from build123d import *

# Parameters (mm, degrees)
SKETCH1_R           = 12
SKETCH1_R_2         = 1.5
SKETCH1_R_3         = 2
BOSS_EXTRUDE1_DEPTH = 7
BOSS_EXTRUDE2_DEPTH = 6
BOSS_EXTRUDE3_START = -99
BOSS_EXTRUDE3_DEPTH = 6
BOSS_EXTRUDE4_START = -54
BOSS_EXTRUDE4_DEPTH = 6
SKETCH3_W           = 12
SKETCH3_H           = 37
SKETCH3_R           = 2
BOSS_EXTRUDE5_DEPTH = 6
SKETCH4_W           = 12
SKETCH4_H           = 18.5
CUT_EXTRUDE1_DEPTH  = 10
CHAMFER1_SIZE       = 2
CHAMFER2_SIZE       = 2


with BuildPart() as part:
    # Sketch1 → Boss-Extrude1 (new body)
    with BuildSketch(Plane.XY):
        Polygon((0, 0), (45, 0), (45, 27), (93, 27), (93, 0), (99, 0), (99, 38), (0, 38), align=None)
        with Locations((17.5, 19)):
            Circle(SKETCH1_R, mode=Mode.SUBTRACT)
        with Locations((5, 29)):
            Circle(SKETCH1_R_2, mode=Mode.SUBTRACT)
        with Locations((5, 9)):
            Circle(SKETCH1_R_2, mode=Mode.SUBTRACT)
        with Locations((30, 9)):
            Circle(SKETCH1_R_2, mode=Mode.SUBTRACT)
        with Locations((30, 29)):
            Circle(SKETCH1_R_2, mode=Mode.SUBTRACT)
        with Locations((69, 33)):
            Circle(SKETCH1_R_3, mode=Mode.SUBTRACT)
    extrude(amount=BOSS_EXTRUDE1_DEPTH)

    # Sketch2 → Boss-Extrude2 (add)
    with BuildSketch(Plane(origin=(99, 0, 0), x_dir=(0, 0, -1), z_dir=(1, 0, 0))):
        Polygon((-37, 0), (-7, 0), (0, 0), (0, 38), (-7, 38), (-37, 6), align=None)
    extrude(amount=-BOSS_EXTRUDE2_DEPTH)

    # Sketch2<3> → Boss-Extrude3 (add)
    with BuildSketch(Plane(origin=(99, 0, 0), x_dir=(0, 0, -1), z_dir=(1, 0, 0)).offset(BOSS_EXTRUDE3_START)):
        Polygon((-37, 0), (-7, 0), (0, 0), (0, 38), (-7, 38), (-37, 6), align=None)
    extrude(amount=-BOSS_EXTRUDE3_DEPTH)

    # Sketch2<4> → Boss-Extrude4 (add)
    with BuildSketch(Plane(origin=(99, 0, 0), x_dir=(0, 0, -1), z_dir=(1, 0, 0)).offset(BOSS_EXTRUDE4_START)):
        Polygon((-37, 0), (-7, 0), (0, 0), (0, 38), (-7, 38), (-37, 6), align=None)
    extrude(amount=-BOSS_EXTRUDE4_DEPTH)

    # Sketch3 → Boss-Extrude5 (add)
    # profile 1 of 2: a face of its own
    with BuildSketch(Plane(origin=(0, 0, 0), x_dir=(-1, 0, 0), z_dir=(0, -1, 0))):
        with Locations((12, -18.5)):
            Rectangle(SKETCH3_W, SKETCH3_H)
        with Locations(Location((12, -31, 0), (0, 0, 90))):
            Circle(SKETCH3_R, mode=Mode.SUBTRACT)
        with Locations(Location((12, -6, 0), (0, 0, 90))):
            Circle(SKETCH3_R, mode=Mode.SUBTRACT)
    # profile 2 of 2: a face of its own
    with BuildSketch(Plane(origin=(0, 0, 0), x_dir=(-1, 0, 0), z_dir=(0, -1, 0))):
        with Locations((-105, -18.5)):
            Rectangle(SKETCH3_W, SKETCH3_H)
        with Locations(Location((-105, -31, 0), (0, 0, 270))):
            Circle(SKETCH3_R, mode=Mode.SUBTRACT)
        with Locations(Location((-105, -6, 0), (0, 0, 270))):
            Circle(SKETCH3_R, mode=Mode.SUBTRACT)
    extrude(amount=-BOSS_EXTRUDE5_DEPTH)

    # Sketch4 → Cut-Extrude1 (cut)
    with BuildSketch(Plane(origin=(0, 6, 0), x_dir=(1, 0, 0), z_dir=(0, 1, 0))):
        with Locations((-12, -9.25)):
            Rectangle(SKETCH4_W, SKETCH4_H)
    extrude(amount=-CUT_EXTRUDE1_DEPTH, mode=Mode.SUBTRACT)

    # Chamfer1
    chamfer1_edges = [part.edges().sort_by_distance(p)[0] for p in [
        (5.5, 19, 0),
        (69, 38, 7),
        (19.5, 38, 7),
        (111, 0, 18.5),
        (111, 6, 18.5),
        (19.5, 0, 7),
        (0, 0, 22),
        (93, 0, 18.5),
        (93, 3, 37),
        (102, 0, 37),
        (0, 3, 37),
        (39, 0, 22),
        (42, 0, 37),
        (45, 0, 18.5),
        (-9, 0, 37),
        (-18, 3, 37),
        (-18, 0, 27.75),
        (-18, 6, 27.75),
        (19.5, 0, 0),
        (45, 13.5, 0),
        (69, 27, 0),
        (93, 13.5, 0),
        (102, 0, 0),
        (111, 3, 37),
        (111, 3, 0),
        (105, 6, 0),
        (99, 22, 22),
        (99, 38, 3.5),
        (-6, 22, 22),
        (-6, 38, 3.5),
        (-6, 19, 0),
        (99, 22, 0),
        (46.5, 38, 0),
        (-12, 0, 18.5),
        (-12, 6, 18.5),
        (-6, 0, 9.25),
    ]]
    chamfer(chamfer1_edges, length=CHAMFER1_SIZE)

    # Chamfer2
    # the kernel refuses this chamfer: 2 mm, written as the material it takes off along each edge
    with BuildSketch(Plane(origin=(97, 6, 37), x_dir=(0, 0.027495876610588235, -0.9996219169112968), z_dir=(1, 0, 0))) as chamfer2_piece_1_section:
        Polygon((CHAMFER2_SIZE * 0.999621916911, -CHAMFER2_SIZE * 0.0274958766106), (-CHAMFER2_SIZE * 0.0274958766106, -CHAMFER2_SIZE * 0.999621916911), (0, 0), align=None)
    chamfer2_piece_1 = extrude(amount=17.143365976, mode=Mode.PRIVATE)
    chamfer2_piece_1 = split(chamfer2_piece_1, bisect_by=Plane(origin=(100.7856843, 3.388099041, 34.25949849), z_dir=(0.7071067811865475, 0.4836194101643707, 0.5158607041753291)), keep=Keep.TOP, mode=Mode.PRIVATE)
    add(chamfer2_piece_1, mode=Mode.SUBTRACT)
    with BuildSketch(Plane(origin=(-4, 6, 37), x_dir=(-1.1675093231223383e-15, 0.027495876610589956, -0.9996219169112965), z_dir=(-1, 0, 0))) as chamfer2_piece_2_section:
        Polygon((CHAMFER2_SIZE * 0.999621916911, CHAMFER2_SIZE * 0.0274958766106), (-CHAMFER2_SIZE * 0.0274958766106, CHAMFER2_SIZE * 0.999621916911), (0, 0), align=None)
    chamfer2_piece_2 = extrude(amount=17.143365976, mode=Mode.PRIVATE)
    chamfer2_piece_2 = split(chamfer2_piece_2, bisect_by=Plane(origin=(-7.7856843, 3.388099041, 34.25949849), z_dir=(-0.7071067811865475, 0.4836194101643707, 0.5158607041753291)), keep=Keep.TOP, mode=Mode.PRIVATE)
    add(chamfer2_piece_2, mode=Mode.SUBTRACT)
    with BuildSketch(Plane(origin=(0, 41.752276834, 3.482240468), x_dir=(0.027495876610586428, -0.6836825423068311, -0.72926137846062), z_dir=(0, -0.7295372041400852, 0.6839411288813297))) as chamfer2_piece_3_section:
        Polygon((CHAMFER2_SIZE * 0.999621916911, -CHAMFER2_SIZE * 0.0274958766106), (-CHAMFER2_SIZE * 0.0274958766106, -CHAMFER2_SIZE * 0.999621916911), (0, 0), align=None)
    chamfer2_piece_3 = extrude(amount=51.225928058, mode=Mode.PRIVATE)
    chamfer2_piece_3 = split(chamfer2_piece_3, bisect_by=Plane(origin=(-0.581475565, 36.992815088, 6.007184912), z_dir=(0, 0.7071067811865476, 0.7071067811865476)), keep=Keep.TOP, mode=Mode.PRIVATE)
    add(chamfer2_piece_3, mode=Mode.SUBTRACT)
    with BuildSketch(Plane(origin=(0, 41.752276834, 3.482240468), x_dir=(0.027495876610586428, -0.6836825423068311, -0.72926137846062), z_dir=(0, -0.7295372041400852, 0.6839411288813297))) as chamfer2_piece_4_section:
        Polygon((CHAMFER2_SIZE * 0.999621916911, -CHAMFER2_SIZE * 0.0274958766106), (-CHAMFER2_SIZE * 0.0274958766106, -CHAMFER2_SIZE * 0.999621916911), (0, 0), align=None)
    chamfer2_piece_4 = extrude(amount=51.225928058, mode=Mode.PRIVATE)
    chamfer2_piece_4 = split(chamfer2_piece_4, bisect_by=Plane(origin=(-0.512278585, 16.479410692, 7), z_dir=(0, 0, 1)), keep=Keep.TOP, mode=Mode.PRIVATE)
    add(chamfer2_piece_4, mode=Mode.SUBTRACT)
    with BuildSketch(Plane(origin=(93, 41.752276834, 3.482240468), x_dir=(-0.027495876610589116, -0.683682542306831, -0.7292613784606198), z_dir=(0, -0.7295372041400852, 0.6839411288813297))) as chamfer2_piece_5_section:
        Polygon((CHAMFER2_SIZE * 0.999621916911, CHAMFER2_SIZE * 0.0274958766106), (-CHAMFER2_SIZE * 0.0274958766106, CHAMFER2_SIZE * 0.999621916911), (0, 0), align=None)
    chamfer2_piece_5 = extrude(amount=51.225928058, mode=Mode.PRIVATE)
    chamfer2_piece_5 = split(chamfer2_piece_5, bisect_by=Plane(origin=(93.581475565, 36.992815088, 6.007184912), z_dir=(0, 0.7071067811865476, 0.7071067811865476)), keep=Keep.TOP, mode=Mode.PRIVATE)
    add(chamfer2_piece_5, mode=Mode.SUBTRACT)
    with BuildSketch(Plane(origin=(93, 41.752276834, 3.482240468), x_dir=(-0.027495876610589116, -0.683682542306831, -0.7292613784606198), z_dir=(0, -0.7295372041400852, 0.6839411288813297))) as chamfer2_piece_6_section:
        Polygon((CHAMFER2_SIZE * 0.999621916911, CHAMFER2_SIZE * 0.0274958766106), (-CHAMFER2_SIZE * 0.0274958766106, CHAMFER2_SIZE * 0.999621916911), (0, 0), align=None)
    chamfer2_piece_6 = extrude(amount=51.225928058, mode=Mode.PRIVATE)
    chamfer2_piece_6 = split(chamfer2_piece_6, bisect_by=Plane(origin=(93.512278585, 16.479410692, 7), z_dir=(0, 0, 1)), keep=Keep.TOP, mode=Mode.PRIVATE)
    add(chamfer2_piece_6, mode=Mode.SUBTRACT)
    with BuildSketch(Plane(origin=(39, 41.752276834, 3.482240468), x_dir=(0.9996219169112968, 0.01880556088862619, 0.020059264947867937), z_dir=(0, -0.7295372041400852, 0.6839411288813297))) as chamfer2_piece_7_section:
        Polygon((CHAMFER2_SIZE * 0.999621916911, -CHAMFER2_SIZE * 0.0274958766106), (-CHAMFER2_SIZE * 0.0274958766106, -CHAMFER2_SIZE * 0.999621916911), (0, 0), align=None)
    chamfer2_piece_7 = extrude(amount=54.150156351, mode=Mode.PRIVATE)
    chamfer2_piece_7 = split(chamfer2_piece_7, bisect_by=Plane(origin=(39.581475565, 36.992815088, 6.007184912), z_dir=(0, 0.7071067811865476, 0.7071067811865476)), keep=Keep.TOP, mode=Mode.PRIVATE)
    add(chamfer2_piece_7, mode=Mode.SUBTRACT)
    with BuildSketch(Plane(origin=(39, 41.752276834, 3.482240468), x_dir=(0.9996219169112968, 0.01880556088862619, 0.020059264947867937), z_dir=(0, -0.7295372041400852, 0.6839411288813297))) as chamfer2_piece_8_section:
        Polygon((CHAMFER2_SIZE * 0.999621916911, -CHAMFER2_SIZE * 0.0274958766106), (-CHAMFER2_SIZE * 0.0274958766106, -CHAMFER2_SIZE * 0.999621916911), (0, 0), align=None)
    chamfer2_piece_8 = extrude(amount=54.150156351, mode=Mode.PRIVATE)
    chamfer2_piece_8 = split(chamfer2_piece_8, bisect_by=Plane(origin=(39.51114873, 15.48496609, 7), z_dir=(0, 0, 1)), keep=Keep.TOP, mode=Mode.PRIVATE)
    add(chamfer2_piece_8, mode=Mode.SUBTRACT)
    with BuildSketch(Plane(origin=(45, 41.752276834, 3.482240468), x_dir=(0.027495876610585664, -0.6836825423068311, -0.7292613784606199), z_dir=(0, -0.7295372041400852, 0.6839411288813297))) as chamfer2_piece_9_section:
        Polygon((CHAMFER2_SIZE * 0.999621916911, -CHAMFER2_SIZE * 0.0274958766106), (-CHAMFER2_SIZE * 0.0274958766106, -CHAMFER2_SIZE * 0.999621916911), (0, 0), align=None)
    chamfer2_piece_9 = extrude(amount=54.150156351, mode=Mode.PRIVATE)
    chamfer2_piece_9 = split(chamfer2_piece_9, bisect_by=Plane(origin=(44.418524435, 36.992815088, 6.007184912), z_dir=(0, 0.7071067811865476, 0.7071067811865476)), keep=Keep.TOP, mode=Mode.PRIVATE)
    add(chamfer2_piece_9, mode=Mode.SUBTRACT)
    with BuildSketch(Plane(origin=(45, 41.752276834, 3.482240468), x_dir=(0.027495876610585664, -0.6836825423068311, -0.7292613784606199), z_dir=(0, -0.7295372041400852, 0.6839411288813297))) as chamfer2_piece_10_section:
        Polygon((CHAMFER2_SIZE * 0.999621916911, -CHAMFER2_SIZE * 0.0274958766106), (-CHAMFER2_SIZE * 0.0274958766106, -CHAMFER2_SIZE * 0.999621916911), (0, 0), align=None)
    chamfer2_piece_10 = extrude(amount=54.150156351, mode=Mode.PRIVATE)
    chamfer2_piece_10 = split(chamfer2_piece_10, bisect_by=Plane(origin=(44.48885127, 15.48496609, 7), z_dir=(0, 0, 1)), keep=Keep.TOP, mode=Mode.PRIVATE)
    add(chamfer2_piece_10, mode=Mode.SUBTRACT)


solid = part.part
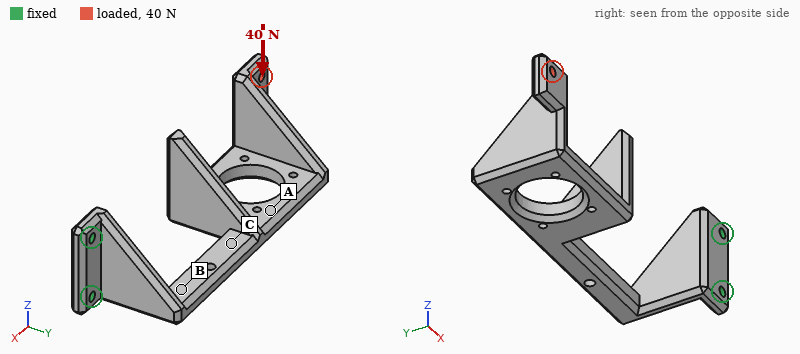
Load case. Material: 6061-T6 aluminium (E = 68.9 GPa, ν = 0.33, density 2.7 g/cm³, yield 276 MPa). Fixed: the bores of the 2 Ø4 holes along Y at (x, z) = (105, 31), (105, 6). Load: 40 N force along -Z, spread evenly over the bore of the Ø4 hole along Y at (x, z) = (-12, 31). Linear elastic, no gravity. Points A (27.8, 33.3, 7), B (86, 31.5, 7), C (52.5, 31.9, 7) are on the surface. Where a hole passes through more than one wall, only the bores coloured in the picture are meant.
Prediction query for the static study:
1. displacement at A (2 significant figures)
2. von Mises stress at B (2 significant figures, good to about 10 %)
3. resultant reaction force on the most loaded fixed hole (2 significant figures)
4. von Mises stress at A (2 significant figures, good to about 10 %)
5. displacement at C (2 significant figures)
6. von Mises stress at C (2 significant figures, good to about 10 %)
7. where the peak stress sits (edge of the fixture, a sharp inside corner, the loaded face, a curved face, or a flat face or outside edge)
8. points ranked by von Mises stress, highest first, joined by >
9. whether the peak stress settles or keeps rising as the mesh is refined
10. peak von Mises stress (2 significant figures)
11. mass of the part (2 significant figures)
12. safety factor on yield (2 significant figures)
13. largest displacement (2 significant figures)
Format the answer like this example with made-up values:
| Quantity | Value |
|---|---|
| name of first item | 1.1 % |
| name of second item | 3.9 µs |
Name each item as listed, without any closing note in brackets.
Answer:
| Quantity | Value |
|---|---|
| displacement at A | 0.70 mm |
| von Mises stress at B | 52 MPa |
| resultant reaction force on the most loaded fixed hole | 190 N |
| von Mises stress at A | 12 MPa |
| displacement at C | 0.37 mm |
| von Mises stress at C | 37 MPa |
| where the peak stress sits | a curved face |
| points ranked by von Mises stress, highest first, joined by > | B > C > A |
| whether the peak stress settles or keeps rising as the mesh is refined | settles |
| peak von Mises stress | 130 MPa |
| mass of the part | 77 g |
| safety factor on yield | 2.1 |
| largest displacement | 1.6 mm |
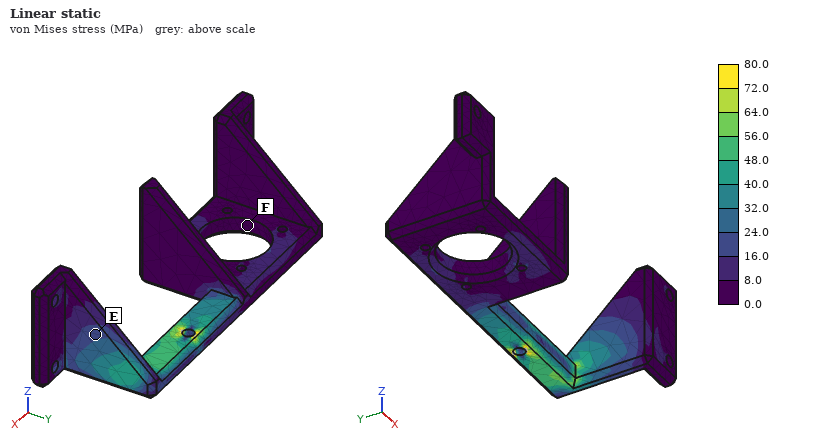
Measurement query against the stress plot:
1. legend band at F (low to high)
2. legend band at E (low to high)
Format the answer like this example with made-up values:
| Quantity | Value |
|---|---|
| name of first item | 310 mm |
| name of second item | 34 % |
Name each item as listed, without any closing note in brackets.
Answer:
| Quantity | Value |
|---|---|
| legend band at F | 0.0 to 8.0 MPa |
| legend band at E | 16.0 to 24.0 MPa |
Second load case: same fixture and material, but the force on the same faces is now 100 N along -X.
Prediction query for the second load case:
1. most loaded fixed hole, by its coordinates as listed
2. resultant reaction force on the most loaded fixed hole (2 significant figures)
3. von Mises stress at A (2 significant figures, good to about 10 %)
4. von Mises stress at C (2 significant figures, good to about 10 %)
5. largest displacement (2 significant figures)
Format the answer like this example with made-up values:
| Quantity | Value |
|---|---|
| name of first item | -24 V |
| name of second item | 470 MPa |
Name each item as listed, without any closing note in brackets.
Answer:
| Quantity | Value |
|---|---|
| most loaded fixed hole, by its coordinates as listed | (105, 31) |
| resultant reaction force on the most loaded fixed hole | 100 N |
| von Mises stress at A | 23 MPa |
| von Mises stress at C | 37 MPa |
| largest displacement | 1.4 mm |
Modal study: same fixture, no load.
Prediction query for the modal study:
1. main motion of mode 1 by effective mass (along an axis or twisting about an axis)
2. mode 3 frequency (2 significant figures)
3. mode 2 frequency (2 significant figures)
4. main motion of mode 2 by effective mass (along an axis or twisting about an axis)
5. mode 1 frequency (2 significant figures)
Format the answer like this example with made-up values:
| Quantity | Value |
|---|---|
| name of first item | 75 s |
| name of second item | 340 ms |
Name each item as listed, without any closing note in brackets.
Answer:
| Quantity | Value |
|---|---|
| main motion of mode 1 by effective mass | along Z |
| mode 3 frequency | 800 Hz |
| mode 2 frequency | 190 Hz |
| main motion of mode 2 by effective mass | along Y |
| mode 1 frequency | 170 Hz |
